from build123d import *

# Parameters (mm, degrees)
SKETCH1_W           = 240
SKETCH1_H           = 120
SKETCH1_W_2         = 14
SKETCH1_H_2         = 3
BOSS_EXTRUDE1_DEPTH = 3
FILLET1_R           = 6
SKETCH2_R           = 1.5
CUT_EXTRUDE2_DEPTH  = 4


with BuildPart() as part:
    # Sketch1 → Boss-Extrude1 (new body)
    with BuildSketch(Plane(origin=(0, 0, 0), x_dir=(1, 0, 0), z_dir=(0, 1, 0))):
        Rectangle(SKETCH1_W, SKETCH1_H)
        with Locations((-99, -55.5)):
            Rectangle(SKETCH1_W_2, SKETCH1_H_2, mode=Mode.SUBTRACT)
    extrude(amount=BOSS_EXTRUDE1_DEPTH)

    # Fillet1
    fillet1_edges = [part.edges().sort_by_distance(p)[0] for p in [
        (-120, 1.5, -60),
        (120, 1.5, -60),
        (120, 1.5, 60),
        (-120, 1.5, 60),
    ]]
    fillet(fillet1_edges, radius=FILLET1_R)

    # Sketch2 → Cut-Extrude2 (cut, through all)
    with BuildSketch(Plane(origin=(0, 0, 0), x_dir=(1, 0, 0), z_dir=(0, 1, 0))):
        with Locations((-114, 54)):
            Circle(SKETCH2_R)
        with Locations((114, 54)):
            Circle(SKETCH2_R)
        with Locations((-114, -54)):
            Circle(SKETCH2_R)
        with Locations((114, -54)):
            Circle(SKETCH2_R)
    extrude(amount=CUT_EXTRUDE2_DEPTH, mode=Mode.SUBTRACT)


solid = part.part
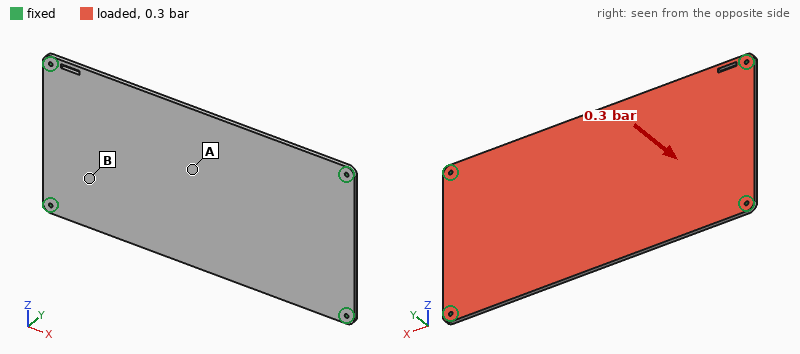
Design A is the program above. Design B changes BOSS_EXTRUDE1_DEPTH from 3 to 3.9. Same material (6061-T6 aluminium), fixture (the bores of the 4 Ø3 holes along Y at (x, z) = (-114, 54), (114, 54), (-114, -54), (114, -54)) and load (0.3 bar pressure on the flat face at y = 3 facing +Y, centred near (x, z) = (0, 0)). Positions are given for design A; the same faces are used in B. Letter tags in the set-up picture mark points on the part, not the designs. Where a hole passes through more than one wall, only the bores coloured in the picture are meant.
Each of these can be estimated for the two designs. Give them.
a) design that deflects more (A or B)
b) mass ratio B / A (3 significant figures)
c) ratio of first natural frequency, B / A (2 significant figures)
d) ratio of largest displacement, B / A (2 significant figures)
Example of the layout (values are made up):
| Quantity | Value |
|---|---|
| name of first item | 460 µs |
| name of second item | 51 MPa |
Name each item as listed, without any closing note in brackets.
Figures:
| Quantity | Value |
|---|---|
| design that deflects more | A |
| mass ratio B / A | 1.30 |
| ratio of first natural frequency, B / A | 1.3 |
| ratio of largest displacement, B / A | 0.47 |
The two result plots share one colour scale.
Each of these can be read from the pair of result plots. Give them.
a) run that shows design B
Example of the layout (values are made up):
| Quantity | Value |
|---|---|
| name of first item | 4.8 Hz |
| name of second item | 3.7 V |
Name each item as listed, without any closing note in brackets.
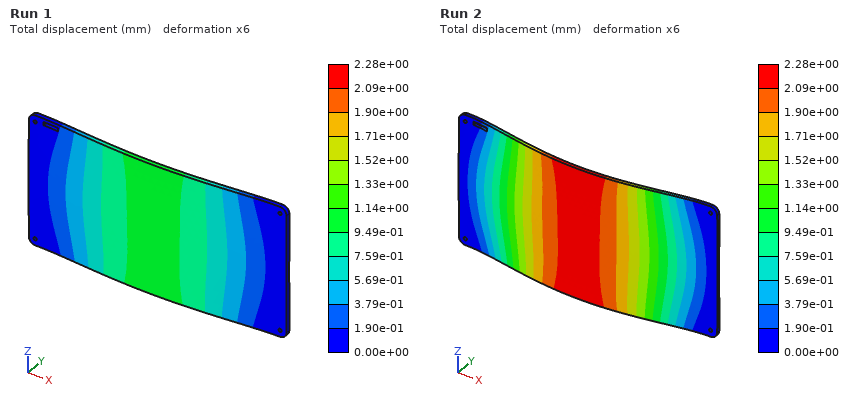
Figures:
| Quantity | Value |
|---|---|
| run that shows design B | Run 1 |
